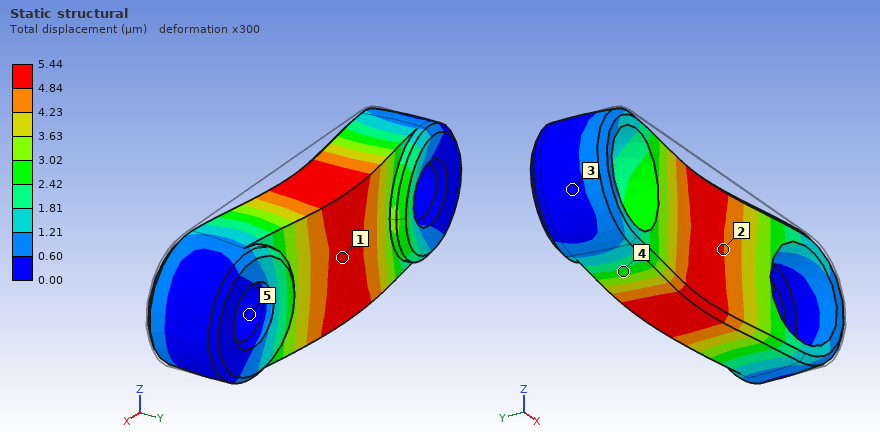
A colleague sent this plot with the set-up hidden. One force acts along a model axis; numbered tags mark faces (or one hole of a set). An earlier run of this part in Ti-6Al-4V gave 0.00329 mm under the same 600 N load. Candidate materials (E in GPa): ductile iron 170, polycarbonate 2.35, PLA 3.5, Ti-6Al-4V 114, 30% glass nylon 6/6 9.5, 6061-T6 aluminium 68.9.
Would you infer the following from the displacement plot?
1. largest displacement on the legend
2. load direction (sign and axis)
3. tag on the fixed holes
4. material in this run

5.44 µm
+Y
5
6061-T6 aluminium
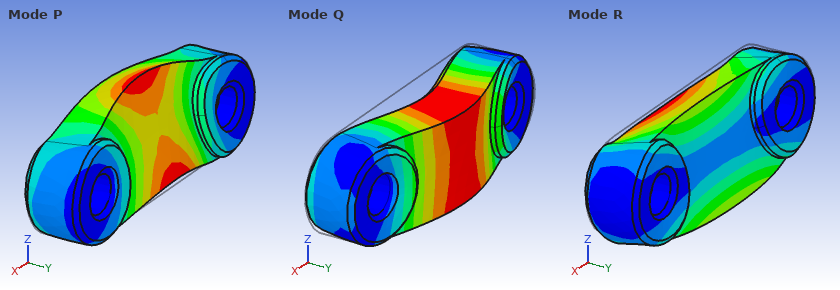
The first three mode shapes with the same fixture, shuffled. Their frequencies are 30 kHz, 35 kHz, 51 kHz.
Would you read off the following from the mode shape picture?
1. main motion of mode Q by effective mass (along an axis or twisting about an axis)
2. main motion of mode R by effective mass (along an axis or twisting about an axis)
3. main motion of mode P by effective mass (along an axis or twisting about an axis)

along Y
along Z
along Z
